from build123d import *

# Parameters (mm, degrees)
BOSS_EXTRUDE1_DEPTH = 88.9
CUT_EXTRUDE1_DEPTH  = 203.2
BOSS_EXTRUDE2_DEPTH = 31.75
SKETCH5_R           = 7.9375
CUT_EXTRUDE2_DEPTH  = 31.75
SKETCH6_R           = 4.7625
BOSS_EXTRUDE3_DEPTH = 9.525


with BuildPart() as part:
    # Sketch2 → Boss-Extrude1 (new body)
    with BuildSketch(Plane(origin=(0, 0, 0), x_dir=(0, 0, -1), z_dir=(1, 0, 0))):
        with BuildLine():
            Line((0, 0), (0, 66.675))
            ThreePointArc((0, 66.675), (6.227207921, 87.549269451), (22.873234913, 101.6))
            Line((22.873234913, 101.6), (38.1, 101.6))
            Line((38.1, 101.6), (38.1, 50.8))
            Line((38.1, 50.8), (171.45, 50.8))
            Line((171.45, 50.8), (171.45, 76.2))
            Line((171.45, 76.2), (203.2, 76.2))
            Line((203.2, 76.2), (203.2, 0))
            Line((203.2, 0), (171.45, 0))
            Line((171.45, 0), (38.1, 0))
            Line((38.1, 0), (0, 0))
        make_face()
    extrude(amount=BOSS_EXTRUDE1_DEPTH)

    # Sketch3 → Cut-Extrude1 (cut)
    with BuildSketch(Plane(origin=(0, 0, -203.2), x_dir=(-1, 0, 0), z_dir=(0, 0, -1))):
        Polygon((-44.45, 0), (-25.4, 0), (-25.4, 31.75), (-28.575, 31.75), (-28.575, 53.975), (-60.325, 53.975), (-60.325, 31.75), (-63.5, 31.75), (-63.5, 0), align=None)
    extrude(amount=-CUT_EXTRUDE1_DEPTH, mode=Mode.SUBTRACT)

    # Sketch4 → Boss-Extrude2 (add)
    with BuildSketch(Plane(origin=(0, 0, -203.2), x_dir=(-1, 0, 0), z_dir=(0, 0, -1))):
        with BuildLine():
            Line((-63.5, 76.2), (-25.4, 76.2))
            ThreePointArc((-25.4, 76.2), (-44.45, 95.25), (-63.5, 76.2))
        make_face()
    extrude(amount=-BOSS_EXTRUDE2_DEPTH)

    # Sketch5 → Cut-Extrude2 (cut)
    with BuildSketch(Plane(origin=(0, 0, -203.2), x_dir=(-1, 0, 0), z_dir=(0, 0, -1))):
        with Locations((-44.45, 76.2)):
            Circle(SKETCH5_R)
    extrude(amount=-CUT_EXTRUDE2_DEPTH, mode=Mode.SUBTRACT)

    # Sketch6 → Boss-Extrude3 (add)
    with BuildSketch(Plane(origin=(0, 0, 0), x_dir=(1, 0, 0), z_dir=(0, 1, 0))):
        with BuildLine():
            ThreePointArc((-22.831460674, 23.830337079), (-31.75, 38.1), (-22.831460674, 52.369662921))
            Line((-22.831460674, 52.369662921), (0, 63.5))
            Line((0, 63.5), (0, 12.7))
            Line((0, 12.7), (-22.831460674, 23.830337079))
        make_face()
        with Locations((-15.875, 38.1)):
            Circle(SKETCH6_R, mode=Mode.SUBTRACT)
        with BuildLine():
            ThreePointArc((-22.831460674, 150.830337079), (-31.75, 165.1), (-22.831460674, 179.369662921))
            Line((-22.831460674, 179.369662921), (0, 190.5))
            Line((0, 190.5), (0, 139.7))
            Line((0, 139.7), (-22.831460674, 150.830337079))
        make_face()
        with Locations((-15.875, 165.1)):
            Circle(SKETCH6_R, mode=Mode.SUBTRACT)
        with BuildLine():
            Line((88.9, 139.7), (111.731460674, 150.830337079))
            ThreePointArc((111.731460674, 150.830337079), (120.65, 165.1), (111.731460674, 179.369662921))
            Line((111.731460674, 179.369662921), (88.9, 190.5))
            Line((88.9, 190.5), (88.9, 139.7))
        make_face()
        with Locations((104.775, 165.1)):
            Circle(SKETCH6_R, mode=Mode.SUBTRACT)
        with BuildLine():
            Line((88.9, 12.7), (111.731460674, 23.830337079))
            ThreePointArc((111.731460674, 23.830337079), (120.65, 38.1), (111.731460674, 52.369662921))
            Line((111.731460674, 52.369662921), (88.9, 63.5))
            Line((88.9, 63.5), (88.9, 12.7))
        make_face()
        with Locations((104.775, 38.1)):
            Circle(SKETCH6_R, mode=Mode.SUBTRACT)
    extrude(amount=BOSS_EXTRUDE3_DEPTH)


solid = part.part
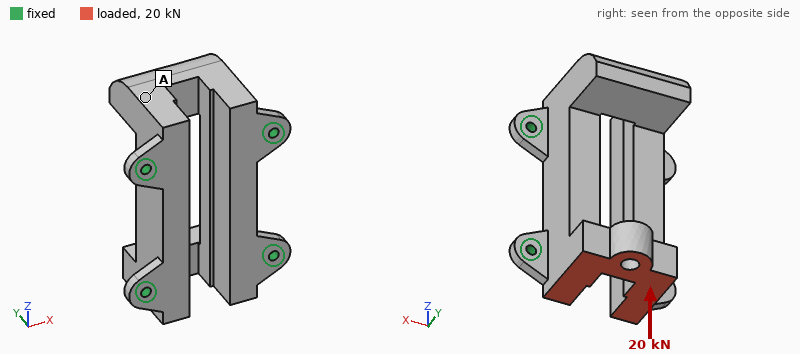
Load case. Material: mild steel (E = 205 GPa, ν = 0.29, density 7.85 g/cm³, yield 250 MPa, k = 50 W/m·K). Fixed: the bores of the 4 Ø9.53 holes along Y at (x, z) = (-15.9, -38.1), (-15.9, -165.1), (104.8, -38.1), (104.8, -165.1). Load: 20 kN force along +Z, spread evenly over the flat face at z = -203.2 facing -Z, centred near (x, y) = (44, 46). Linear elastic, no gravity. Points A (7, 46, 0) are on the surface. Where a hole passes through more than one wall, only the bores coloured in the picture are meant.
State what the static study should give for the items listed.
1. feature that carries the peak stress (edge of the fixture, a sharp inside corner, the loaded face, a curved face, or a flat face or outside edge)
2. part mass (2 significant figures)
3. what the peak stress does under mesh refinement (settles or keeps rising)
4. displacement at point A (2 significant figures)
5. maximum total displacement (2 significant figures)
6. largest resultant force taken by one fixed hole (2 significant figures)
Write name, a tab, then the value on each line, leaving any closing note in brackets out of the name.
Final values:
feature that carries the peak stress	edge of the fixture
part mass	6.4 kg
what the peak stress does under mesh refinement	keeps rising
displacement at point A	14 µm
maximum total displacement	51 µm
largest resultant force taken by one fixed hole	6.8 kN
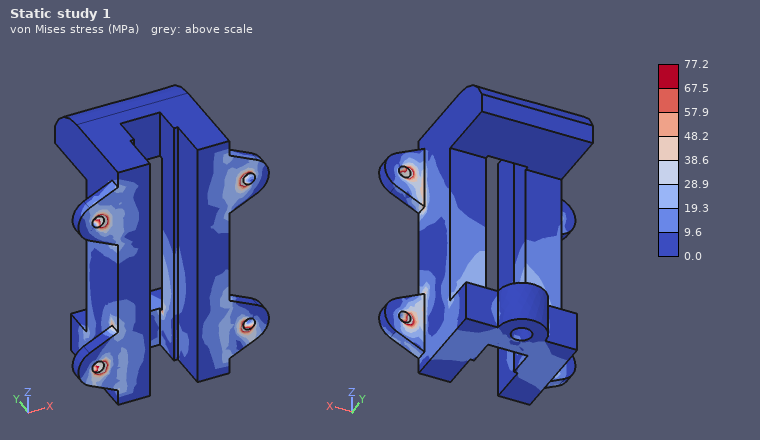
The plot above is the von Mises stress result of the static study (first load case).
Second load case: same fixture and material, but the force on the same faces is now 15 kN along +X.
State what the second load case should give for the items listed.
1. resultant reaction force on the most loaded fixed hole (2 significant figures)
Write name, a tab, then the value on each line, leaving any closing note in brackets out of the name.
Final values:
resultant reaction force on the most loaded fixed hole	9.9 kN
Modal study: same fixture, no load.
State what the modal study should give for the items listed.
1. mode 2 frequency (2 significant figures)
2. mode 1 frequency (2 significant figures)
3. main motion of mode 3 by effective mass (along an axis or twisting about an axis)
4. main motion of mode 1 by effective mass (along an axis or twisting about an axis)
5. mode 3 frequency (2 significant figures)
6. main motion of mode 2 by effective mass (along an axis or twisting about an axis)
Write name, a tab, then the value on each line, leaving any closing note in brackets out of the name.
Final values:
mode 2 frequency	2400 Hz
mode 1 frequency	1900 Hz
main motion of mode 3 by effective mass	along Y
main motion of mode 1 by effective mass	along Z
mode 3 frequency	2600 Hz
main motion of mode 2 by effective mass	along X
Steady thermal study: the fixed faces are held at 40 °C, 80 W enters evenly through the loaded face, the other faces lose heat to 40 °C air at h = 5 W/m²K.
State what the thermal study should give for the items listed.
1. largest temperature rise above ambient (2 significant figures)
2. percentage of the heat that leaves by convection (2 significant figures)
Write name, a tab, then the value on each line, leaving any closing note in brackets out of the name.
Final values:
largest temperature rise above ambient	60 K
percentage of the heat that leaves by convection	13 %
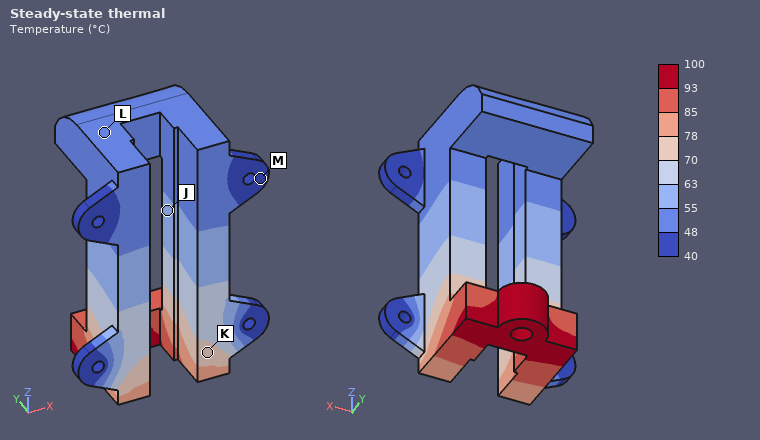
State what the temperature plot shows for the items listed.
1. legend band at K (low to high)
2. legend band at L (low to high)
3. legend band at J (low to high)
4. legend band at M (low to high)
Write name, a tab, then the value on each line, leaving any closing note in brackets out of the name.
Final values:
legend band at K	70 to 78 °C
legend band at L	48 to 55 °C
legend band at J	55 to 63 °C
legend band at M	40 to 48 °C
